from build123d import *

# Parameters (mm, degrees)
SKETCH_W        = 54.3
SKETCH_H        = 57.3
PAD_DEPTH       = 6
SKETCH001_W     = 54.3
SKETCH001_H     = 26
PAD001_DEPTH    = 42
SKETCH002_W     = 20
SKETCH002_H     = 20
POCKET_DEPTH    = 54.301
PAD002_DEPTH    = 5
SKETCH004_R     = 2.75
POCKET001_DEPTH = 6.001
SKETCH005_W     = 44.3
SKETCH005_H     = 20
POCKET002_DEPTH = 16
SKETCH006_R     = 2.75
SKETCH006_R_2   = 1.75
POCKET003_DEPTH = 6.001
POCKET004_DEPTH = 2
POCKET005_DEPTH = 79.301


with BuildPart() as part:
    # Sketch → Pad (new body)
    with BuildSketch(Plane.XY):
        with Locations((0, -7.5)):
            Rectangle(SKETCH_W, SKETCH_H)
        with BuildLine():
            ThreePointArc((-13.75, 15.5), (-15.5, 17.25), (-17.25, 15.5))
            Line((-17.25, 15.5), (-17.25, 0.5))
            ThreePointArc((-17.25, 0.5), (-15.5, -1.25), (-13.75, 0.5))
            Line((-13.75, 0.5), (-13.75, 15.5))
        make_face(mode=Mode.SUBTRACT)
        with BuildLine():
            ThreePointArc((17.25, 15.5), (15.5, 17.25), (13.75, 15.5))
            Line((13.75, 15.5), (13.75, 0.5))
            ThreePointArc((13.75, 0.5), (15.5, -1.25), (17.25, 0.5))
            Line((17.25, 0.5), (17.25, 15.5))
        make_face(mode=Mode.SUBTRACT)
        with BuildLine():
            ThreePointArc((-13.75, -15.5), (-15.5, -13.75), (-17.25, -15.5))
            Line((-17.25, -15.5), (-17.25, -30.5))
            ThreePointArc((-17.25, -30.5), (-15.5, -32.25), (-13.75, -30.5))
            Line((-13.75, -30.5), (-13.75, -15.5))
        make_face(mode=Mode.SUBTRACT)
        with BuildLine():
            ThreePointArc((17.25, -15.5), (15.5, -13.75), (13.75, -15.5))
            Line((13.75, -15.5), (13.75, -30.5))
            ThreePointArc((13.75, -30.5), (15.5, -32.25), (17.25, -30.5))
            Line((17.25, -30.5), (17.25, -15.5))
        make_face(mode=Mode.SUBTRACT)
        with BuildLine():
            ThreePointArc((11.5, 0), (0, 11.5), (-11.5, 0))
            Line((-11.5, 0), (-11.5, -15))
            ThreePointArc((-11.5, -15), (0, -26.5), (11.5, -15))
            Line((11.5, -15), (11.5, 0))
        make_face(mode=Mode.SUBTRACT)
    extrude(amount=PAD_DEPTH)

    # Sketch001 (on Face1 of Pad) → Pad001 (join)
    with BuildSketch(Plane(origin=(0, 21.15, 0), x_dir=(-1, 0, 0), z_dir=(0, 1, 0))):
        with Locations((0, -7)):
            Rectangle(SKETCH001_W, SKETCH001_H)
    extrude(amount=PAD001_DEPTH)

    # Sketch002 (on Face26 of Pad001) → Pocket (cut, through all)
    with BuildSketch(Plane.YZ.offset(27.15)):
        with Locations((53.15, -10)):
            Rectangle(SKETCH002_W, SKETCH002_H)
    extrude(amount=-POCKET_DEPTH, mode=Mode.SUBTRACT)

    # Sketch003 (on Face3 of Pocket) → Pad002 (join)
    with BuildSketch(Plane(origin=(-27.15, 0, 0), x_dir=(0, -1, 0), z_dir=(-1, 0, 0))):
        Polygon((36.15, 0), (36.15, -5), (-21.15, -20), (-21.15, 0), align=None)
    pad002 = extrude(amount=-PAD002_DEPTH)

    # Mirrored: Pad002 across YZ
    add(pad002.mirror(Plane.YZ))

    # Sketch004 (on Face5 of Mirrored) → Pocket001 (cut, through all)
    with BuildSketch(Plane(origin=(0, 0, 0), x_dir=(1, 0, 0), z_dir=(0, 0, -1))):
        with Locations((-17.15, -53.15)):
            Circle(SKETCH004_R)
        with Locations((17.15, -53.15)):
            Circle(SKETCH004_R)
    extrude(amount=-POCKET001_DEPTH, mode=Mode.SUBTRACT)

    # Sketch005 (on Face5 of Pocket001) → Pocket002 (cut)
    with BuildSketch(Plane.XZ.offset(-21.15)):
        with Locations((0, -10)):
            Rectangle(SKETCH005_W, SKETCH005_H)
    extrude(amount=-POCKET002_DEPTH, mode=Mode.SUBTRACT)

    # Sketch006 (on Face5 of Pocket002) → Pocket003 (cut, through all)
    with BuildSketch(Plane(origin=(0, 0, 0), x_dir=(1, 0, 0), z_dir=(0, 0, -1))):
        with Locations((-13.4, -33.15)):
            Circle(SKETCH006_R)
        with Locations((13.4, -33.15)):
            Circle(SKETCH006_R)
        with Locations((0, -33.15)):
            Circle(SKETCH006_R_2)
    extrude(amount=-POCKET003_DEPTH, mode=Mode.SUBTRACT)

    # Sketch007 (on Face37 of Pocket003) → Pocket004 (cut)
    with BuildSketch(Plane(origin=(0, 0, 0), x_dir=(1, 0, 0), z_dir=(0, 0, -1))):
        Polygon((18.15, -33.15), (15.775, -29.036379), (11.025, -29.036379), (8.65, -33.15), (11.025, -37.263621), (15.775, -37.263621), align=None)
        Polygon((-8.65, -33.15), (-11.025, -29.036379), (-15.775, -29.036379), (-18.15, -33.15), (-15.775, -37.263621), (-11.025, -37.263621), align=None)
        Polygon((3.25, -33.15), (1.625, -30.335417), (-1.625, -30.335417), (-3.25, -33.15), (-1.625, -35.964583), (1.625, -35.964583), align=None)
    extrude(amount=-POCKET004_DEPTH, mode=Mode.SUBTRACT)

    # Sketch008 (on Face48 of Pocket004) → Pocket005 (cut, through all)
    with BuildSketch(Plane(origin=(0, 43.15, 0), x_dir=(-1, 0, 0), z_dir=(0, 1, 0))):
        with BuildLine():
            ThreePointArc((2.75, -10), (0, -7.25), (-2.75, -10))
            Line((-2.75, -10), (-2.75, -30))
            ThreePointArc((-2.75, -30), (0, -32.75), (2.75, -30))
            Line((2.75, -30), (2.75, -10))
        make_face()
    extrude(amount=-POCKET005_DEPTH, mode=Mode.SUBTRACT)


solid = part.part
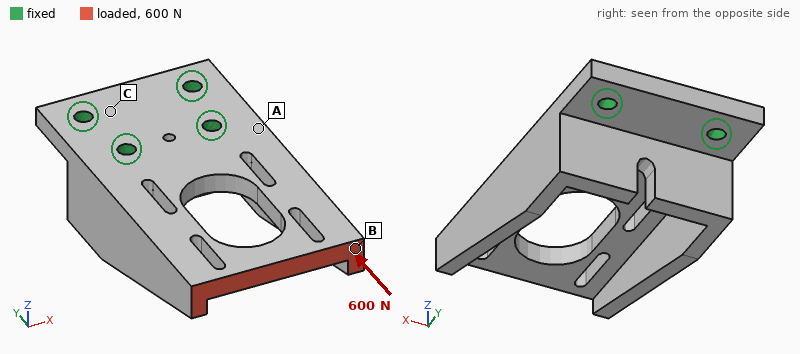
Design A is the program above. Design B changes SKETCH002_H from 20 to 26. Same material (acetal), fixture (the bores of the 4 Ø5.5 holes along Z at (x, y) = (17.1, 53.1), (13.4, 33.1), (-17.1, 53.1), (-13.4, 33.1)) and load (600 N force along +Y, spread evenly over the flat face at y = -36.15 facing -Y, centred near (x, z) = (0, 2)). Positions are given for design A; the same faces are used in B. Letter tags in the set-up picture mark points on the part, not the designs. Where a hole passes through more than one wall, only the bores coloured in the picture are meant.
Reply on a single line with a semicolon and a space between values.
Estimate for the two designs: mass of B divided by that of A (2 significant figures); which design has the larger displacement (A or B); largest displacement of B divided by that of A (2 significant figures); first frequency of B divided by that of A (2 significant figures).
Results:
0.93; A; 0.87; 0.84
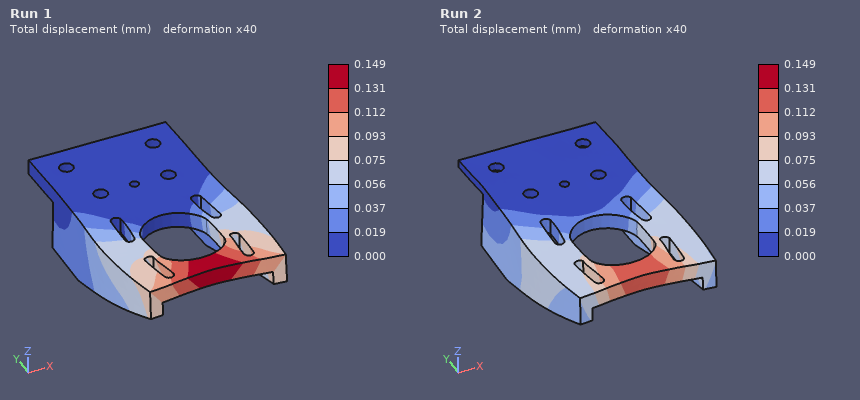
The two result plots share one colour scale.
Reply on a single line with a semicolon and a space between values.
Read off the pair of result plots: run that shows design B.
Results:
Run 2
